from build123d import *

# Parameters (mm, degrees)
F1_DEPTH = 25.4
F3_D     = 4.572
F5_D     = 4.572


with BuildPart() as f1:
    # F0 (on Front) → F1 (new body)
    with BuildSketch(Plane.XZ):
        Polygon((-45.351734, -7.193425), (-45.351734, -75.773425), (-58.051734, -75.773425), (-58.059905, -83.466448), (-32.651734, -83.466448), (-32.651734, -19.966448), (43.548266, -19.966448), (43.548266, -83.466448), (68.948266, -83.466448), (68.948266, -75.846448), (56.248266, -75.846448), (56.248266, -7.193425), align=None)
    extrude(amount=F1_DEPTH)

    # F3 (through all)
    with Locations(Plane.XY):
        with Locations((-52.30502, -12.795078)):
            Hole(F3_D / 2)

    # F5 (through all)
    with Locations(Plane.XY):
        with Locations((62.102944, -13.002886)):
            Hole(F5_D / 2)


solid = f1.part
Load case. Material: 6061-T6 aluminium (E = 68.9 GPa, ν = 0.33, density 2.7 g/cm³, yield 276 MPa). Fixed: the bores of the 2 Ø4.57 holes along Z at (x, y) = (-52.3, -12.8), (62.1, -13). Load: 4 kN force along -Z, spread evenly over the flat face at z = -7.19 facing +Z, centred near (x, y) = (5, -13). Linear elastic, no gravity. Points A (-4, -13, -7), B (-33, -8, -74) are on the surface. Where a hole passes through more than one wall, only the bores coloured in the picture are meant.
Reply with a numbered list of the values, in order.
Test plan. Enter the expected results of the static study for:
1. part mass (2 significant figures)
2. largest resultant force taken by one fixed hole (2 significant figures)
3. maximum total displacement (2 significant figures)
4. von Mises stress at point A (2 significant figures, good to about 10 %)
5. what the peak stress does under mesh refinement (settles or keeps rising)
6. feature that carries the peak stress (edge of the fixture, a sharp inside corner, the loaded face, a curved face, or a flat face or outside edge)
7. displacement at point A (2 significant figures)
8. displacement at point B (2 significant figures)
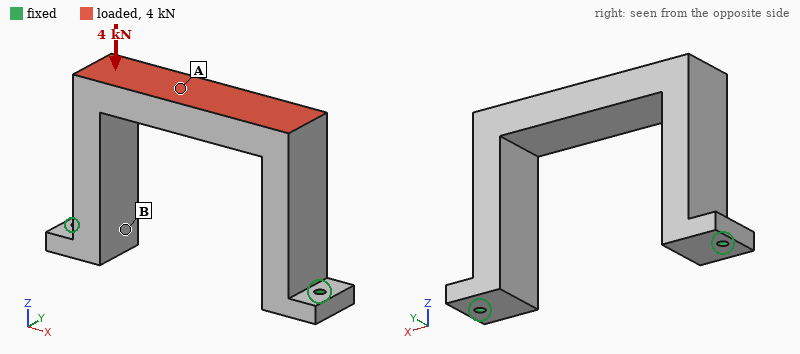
1. 210 g
2. 2.1 kN
3. 55 µm
4. 23 MPa
5. keeps rising
6. edge of the fixture
7. 51 µm
8. 13 µm
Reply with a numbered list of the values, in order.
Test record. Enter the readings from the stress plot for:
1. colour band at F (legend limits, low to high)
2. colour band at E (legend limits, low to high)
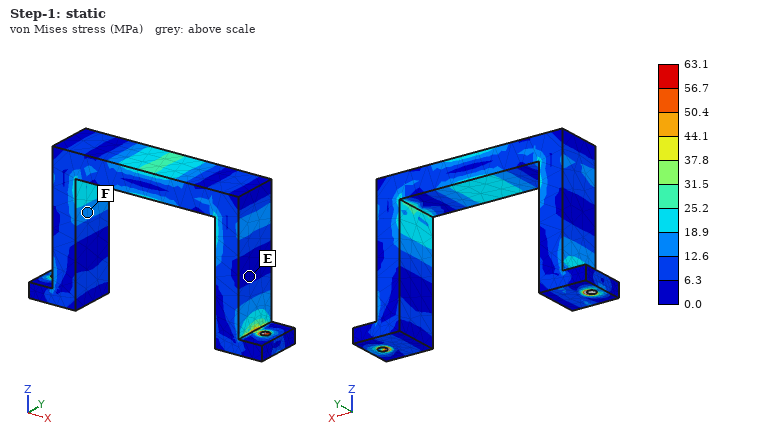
1. 12.6 to 18.9 MPa
2. 0.0 to 6.3 MPa
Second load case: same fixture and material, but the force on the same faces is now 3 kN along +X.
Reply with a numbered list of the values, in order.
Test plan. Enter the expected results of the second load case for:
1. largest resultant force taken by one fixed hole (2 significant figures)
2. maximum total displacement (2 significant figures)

1. 2.2 kN
2. 0.33 mm
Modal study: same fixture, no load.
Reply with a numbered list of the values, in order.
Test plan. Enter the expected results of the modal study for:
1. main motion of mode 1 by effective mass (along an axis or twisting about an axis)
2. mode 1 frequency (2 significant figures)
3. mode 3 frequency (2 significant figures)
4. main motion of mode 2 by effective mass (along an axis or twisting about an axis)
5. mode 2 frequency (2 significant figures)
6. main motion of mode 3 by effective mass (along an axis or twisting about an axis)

1. along Y
2. 850 Hz
3. 2000 Hz
4. along X
5. 1400 Hz
6. twisting about Z
